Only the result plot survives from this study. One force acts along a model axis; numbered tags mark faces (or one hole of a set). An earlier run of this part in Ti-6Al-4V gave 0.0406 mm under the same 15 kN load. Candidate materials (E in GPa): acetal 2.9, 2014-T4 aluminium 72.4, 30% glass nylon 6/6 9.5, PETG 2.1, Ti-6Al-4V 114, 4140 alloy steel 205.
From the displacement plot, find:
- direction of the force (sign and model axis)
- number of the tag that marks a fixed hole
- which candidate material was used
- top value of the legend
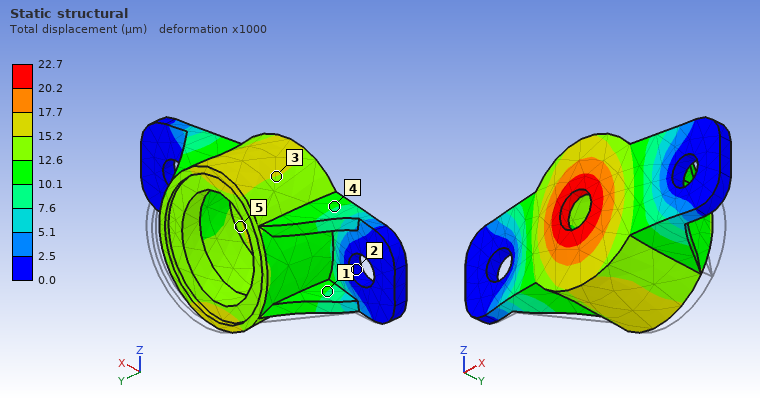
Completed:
-Y
2
4140 alloy steel
22.7 µm
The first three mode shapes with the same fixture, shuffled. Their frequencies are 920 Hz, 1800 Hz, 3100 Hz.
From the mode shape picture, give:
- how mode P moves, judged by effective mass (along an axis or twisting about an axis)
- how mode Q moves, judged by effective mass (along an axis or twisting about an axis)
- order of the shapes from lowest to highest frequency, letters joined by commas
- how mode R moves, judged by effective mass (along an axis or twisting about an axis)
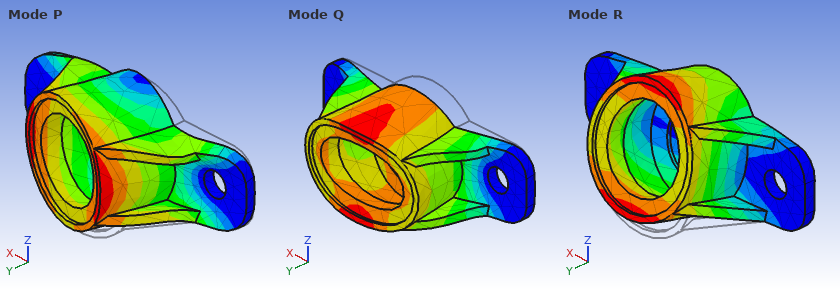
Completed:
along X
along Y
R, Q, P
along Z
